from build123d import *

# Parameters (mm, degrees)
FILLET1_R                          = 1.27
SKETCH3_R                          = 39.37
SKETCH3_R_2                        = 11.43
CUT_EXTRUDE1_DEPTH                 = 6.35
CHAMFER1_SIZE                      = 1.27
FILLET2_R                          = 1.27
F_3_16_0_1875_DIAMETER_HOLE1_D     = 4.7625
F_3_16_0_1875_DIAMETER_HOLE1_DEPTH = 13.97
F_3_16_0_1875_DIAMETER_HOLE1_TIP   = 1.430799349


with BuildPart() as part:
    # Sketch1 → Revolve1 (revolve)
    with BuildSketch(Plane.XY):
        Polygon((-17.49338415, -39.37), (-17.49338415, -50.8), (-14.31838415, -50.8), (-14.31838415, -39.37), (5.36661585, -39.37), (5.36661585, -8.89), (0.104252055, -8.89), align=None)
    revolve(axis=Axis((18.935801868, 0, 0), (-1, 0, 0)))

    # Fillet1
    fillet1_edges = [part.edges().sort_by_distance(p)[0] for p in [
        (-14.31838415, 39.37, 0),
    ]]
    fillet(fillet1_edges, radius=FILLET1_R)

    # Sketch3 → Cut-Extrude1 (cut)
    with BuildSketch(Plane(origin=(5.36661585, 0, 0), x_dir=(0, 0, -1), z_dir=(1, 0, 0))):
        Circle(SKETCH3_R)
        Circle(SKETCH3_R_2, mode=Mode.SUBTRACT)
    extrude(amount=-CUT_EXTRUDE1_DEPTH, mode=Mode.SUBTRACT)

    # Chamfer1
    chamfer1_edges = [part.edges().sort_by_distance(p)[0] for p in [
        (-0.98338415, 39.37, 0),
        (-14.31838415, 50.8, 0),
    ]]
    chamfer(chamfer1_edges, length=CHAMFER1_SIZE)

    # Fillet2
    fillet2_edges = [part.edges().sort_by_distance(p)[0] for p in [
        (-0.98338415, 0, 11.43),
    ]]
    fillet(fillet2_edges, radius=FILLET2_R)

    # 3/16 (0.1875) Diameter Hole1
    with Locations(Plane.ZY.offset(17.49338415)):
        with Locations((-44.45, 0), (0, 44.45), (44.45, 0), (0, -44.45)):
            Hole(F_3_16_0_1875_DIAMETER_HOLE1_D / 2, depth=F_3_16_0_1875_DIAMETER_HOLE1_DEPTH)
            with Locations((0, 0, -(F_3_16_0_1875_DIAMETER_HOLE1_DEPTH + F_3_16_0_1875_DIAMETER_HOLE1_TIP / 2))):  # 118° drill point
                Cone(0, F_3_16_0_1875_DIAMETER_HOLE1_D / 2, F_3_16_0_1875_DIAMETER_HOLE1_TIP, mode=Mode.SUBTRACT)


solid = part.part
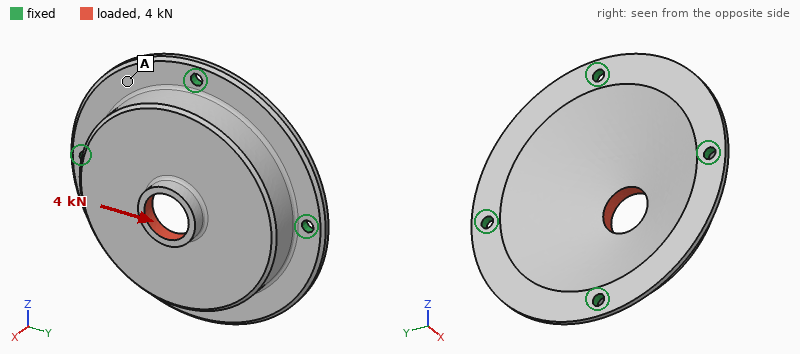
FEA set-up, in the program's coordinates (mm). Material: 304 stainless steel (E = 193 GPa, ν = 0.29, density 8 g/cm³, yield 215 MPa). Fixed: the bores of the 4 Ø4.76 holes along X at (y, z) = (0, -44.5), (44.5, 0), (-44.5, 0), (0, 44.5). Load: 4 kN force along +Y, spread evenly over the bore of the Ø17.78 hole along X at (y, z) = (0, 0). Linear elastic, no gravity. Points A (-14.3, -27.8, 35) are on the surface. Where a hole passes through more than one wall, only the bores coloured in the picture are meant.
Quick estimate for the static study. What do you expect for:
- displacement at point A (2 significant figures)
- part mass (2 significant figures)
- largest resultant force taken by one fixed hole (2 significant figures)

2.9 µm
440 g
1.6 kN
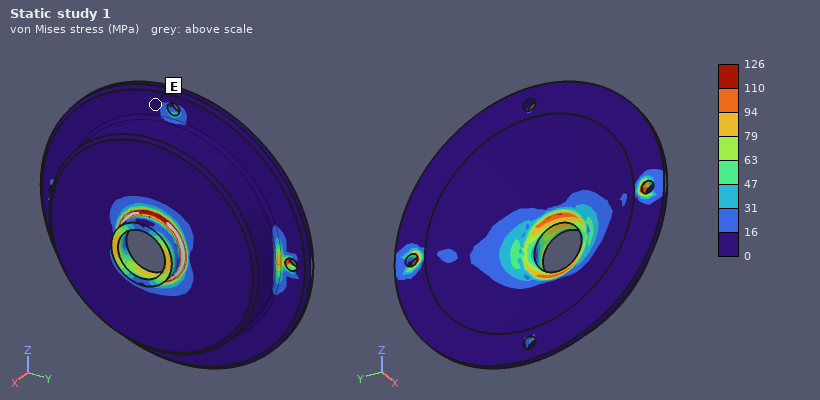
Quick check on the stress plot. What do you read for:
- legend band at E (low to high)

0 to 16 MPa
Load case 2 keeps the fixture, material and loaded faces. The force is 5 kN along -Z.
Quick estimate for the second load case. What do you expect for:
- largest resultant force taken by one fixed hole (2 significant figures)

2.0 kN
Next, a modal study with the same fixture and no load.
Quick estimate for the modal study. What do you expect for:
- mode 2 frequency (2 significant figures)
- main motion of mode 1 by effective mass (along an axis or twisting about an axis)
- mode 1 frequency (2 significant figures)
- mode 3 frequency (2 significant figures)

7400 Hz
along X
7000 Hz
7400 Hz
